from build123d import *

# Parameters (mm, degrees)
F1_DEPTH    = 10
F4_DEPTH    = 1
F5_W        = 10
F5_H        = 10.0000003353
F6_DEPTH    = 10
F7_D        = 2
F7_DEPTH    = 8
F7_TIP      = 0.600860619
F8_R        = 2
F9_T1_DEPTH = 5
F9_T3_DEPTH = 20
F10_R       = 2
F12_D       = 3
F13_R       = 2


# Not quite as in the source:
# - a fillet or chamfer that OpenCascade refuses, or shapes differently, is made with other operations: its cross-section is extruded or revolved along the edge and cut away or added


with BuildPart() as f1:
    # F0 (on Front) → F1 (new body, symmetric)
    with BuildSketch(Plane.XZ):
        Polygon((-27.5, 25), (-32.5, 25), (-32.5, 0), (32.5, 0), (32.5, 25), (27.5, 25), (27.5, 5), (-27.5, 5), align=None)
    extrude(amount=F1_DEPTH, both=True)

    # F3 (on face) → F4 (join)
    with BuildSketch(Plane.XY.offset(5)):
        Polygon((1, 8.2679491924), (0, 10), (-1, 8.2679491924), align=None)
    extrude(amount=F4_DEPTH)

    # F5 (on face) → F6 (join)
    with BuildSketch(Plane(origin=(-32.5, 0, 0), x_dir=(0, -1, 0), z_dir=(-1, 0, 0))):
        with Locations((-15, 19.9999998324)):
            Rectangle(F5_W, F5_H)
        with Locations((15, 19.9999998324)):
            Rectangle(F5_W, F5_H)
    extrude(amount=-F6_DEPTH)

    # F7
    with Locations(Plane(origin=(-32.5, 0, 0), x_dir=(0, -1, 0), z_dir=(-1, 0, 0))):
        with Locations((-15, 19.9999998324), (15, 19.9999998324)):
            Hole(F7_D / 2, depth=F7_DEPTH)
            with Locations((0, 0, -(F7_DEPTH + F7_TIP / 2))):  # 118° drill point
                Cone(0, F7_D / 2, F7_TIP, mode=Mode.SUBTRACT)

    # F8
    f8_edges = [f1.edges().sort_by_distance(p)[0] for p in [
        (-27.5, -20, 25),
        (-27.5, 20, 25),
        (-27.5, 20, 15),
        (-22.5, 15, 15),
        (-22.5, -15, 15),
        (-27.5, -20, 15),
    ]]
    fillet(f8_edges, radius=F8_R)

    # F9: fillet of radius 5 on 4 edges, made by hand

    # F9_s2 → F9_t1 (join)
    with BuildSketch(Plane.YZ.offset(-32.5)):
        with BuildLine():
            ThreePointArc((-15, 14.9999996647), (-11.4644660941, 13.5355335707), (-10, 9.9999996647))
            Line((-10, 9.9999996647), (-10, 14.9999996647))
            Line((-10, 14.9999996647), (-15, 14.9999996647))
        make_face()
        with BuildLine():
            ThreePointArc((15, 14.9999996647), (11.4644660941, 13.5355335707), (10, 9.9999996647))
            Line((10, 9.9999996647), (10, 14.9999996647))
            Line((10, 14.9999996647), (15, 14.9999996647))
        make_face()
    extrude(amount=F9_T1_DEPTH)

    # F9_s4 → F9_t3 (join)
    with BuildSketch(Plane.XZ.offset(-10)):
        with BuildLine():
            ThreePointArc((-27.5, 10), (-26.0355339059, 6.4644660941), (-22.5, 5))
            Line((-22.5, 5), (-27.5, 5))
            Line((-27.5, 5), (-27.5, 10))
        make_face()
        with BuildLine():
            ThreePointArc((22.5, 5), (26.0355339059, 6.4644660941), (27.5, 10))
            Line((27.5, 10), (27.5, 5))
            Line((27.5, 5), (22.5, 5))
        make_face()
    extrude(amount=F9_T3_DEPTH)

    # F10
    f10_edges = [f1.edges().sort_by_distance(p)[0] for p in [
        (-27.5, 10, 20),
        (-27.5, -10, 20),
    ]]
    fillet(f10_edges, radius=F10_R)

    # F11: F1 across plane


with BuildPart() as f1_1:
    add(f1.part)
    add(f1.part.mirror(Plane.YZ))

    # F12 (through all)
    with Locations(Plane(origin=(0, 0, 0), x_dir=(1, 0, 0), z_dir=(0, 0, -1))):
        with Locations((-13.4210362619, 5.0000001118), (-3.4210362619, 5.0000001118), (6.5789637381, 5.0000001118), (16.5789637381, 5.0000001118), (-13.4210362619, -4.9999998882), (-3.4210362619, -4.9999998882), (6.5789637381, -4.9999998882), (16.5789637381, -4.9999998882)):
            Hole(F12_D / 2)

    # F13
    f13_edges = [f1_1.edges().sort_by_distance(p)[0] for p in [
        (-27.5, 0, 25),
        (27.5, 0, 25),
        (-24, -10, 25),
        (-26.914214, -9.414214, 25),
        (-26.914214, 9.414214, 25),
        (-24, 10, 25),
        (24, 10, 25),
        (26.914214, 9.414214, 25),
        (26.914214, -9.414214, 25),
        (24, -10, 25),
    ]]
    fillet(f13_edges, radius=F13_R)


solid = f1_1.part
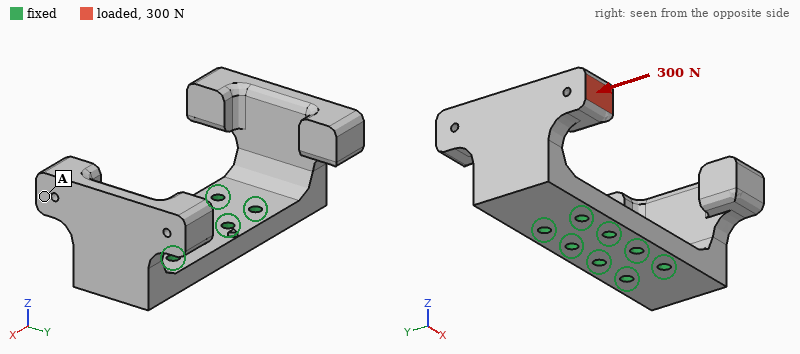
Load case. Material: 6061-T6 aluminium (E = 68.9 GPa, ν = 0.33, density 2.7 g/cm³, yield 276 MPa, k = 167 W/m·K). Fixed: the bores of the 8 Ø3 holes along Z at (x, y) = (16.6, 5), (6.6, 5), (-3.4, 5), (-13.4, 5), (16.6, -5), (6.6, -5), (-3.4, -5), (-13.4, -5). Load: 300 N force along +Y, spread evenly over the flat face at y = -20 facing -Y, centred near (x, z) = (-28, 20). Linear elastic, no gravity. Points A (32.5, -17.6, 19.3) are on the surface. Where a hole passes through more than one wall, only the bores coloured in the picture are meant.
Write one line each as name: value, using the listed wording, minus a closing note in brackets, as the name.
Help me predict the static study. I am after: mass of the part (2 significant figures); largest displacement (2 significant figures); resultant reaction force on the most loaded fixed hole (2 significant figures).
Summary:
mass of the part: 39 g
largest displacement: 85 µm
resultant reaction force on the most loaded fixed hole: 490 N
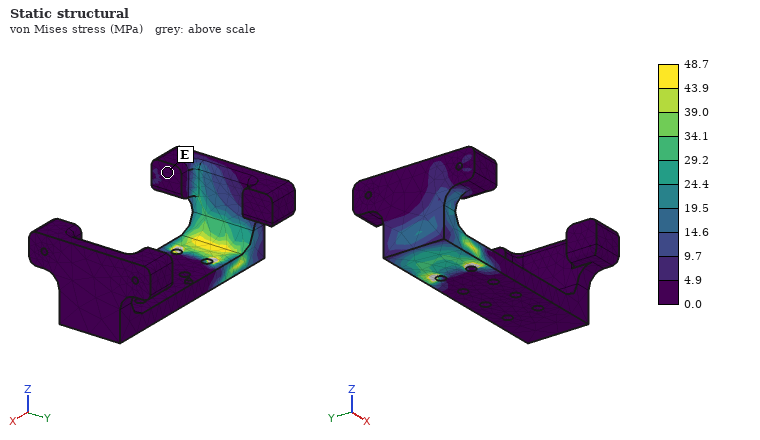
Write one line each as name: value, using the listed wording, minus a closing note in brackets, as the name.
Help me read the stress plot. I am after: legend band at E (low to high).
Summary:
legend band at E: 0.0 to 4.9 MPa
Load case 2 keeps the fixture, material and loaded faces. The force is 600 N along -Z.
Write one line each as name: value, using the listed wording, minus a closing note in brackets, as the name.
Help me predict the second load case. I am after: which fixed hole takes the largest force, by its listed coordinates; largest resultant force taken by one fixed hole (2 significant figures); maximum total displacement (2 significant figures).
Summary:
which fixed hole takes the largest force, by its listed coordinates: (-13.4, -5)
largest resultant force taken by one fixed hole: 1.2 kN
maximum total displacement: 0.24 mm
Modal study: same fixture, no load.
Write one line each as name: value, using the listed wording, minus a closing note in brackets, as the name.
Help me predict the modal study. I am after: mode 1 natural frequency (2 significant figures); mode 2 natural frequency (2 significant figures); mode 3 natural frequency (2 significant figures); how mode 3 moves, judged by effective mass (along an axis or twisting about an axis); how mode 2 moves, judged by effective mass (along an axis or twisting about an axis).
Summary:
mode 1 natural frequency: 2600 Hz
mode 2 natural frequency: 3100 Hz
mode 3 natural frequency: 3500 Hz
how mode 3 moves, judged by effective mass: along Y
how mode 2 moves, judged by effective mass: along X
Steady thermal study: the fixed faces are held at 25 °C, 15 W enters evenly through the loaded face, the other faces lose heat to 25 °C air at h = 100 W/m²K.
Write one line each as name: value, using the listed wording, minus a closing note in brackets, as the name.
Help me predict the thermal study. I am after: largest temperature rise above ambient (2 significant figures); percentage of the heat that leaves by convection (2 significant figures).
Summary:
largest temperature rise above ambient: 36 K
percentage of the heat that leaves by convection: 28 %
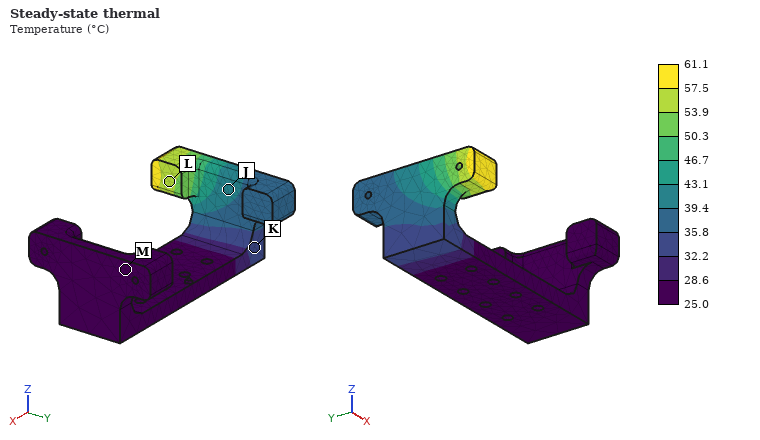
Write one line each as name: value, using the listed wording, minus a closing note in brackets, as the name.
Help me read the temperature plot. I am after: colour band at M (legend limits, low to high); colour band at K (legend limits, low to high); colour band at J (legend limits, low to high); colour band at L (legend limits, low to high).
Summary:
colour band at M: 25.0 to 28.6 °C
colour band at K: 32.2 to 35.8 °C
colour band at J: 39.4 to 43.1 °C
colour band at L: 53.9 to 57.5 °C
